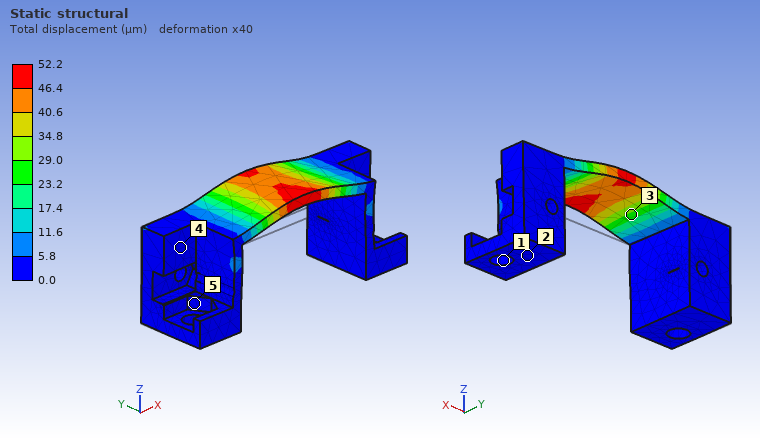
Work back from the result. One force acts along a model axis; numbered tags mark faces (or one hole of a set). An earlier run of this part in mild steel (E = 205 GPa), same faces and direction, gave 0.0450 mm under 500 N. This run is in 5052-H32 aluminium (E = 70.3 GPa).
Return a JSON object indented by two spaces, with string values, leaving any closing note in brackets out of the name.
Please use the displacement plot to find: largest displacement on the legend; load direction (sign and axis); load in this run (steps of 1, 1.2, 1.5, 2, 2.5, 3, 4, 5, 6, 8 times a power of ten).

{
  "largest displacement on the legend": "52.2 µm",
  "load direction": "+Z",
  "load in this run": "200 N"
}
